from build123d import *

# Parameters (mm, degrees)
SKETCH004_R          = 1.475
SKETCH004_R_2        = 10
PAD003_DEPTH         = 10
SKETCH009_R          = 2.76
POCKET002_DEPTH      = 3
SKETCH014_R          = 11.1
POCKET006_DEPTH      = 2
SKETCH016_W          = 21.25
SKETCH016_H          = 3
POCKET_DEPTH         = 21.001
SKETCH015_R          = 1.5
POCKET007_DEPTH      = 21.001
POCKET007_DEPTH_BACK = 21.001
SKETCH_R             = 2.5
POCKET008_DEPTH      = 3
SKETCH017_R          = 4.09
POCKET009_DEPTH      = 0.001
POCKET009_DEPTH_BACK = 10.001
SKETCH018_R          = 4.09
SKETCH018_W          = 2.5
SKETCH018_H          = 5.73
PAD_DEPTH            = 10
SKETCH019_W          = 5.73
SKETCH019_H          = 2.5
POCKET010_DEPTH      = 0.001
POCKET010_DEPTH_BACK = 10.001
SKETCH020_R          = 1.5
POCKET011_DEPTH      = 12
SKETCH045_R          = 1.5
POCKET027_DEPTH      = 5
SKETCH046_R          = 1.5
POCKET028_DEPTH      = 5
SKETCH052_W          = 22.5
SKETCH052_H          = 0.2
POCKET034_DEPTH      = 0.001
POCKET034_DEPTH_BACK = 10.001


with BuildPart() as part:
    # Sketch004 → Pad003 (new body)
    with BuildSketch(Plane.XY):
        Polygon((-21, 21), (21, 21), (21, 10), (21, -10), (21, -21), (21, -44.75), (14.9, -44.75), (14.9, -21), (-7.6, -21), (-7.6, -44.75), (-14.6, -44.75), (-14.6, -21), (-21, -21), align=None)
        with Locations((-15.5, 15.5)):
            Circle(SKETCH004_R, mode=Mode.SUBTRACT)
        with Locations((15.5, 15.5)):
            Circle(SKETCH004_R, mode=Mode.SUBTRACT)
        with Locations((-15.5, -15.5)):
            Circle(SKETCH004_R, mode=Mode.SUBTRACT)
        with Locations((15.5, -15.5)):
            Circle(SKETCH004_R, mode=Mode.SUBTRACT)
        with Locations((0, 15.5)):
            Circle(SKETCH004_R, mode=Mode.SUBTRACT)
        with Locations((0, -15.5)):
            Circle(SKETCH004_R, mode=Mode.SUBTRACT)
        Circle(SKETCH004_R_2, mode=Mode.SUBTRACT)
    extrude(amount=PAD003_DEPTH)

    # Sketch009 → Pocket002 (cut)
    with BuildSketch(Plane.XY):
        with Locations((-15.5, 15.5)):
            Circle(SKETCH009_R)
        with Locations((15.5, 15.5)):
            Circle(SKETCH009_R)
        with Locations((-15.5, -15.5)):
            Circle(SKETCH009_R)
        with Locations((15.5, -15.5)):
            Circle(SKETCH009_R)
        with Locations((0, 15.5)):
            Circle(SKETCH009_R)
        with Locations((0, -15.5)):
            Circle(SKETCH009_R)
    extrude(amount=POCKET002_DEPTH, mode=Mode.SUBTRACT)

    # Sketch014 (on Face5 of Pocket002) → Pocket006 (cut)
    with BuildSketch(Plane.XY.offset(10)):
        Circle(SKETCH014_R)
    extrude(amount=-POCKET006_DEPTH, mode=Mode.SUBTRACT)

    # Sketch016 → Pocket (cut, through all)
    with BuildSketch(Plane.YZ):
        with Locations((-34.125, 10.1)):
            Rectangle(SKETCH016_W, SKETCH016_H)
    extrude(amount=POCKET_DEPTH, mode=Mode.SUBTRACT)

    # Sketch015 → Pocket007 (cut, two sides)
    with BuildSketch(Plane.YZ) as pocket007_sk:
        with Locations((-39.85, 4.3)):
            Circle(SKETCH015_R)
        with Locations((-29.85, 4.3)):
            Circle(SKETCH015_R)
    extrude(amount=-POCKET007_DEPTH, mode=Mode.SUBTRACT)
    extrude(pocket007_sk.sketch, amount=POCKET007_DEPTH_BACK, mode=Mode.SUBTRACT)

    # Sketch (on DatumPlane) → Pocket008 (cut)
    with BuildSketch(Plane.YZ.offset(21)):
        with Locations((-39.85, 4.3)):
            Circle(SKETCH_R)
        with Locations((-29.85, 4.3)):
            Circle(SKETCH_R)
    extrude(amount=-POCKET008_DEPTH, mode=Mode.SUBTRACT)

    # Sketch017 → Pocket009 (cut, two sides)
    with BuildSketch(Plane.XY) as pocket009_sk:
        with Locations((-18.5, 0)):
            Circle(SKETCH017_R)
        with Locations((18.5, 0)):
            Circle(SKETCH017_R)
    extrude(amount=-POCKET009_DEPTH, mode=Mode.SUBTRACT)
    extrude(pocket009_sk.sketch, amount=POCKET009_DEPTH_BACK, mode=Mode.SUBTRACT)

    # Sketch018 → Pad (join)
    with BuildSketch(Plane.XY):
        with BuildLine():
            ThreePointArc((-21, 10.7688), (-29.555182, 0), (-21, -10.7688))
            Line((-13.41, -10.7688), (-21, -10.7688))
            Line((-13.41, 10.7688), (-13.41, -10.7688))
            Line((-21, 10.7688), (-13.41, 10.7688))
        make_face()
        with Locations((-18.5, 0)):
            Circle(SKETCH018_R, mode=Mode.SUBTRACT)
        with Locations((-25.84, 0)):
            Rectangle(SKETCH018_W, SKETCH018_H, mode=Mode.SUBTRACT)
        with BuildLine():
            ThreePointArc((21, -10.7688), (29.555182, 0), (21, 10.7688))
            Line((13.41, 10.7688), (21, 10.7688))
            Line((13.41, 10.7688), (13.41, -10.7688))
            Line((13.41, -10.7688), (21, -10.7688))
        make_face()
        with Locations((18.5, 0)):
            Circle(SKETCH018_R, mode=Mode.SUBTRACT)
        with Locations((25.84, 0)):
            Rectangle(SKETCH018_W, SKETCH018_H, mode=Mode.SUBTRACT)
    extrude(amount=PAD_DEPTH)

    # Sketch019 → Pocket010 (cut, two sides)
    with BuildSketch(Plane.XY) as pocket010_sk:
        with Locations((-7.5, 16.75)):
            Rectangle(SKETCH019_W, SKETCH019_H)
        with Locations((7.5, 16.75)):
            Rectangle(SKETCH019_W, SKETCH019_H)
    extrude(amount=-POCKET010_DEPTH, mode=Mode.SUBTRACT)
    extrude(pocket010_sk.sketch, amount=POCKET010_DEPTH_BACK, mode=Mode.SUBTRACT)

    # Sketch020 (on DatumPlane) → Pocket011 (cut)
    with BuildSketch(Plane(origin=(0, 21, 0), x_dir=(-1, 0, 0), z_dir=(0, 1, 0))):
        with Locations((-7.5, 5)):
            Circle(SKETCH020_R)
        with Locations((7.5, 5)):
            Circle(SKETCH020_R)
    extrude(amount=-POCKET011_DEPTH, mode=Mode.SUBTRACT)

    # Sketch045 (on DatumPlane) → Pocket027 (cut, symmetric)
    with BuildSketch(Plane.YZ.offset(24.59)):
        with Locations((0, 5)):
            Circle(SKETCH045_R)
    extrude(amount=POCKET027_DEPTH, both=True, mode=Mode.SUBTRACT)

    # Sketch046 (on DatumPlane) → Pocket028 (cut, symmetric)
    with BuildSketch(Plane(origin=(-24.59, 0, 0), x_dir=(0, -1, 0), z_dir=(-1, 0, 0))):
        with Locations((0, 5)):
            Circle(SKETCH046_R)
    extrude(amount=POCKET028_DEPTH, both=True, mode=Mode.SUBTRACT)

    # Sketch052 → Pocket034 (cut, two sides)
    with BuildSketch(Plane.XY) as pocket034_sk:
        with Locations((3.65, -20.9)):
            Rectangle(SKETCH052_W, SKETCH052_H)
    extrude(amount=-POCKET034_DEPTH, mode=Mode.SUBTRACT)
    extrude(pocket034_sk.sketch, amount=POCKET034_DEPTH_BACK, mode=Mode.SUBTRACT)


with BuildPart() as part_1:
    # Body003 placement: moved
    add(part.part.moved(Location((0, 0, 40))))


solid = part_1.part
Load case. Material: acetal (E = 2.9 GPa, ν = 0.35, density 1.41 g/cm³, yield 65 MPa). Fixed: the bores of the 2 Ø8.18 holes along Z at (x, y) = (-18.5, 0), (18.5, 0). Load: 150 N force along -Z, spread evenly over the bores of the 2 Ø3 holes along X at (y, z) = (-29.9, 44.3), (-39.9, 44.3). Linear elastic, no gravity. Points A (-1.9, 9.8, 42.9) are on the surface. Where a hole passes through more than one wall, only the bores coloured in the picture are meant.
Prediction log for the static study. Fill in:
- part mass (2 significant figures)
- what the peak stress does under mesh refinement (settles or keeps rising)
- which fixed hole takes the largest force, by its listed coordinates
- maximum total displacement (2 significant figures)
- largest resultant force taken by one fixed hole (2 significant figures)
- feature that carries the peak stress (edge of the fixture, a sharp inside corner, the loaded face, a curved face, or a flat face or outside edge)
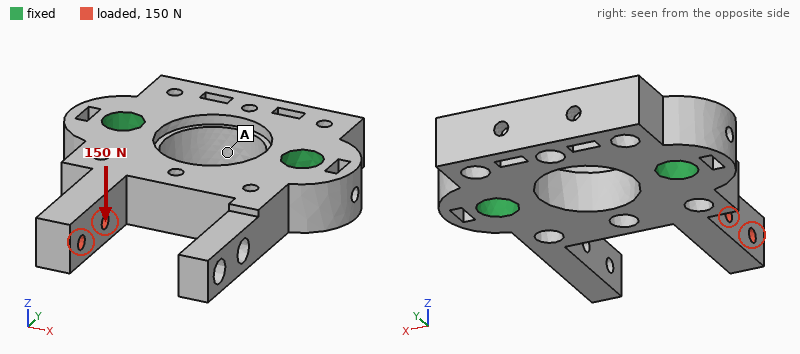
24 g
keeps rising
(-18.5, 0)
0.89 mm
120 N
a sharp inside corner
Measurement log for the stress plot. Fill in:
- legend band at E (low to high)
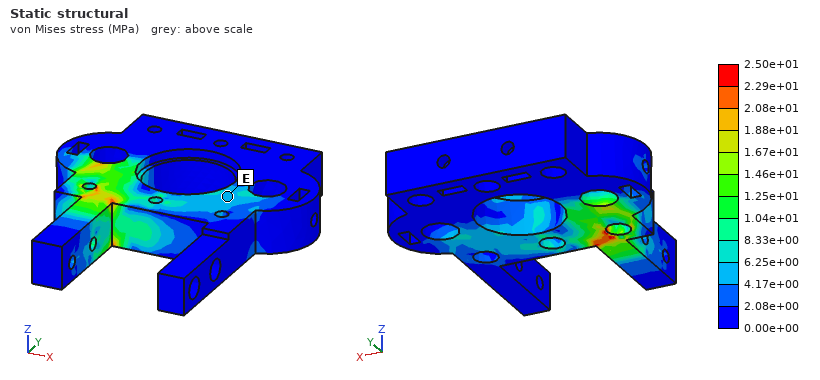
4.17e+00 to 6.25e+00 MPa
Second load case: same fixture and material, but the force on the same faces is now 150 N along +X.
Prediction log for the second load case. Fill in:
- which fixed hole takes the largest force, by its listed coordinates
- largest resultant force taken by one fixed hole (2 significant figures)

(18.5, 0)
170 N
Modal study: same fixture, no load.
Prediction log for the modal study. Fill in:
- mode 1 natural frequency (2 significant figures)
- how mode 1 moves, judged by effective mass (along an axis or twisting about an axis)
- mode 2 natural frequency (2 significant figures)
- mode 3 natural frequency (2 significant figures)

1600 Hz
along Z
1800 Hz
1900 Hz
